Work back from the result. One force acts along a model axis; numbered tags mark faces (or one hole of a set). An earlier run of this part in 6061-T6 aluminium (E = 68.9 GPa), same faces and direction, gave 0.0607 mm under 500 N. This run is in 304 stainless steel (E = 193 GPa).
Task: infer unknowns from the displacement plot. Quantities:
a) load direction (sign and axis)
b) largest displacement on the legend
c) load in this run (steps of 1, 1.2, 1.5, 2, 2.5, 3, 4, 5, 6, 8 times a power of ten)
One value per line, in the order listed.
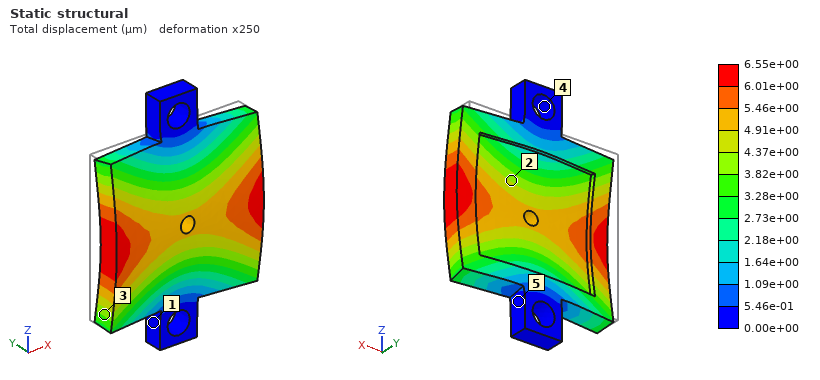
-Y
6.55e+00 µm
150 N
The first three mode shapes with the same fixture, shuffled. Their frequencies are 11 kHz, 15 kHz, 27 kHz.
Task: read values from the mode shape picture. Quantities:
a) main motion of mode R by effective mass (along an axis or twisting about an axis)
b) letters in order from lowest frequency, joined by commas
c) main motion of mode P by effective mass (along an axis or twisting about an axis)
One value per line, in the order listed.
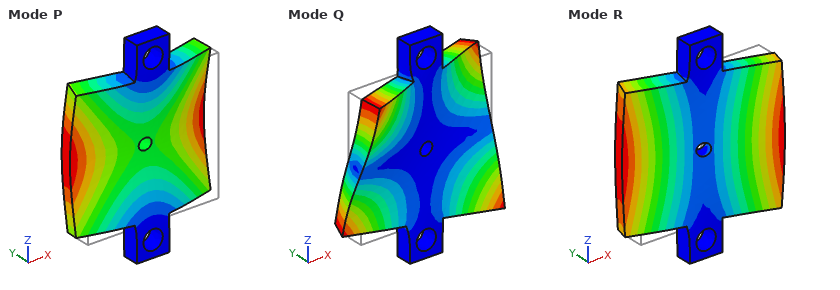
twisting about Z
R, P, Q
along Y
